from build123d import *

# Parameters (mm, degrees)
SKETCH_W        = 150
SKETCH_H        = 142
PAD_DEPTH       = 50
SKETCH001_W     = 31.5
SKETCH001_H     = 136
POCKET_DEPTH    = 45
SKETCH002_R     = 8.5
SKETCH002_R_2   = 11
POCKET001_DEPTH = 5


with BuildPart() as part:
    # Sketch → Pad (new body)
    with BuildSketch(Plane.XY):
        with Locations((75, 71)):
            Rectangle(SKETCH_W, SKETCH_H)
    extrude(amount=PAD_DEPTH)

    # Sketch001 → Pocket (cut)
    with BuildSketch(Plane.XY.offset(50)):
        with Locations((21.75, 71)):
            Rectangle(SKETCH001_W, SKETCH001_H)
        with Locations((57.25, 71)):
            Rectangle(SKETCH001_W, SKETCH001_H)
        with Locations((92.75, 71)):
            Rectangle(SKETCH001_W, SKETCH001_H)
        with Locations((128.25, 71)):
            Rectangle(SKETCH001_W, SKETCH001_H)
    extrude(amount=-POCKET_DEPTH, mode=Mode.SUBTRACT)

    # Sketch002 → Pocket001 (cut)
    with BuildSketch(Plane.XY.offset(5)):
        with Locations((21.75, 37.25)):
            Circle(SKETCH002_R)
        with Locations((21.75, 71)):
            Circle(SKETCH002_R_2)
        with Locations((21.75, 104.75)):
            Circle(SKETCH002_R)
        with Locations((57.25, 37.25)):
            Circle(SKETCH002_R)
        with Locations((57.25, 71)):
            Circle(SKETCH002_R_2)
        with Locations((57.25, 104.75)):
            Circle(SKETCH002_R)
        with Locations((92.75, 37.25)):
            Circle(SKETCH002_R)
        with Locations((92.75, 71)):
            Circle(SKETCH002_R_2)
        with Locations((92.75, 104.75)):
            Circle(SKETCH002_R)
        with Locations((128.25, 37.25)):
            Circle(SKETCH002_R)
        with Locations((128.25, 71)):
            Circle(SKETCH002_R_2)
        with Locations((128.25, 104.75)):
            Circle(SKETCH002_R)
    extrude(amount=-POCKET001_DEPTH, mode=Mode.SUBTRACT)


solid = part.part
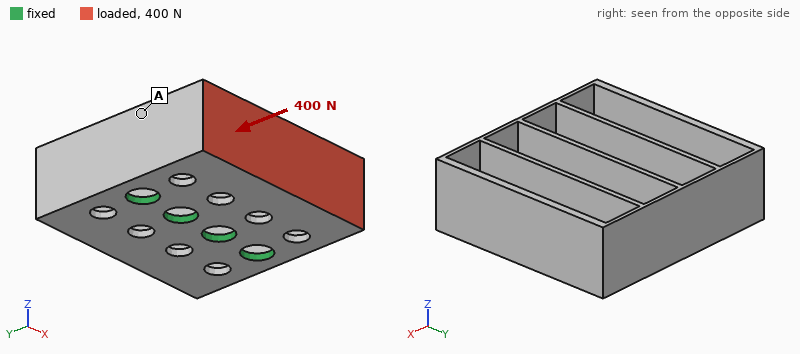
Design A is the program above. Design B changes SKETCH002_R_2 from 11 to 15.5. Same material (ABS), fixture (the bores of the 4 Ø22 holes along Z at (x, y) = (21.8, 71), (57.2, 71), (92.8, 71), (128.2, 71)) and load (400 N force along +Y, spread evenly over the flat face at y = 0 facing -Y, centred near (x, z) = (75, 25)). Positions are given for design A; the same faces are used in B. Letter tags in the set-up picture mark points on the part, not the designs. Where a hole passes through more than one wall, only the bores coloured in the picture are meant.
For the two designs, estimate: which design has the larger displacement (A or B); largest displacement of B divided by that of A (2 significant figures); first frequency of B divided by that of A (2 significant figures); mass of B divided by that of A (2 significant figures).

A
0.57
1.4
0.97
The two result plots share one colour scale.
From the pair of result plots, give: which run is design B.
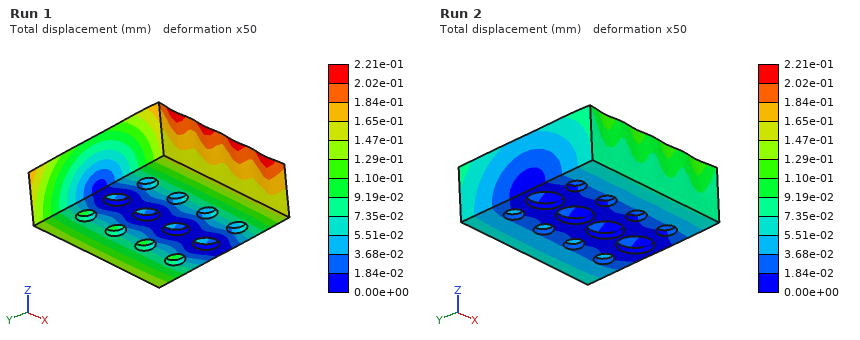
Run 2
